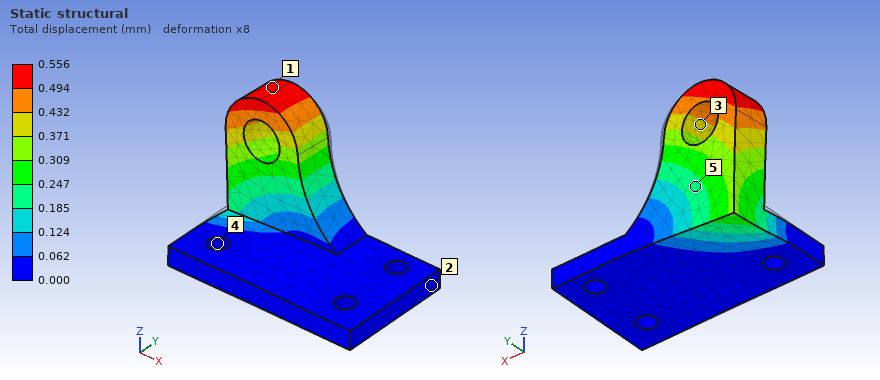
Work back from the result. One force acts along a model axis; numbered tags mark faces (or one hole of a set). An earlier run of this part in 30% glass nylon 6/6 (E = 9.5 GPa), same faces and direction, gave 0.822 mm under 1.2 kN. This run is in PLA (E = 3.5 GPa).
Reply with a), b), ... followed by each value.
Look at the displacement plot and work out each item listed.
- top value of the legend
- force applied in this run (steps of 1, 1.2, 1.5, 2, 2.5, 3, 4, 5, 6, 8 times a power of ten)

a) 0.556 mm
b) 300 N
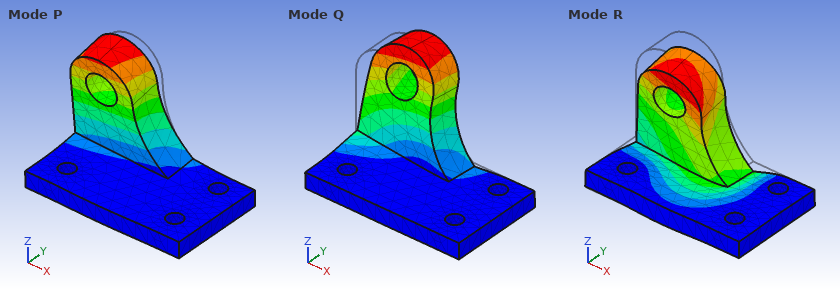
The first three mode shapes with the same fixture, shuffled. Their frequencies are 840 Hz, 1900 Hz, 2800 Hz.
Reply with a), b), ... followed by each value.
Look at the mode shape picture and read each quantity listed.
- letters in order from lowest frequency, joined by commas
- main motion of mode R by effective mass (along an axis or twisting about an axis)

a) P, Q, R
b) along Z
